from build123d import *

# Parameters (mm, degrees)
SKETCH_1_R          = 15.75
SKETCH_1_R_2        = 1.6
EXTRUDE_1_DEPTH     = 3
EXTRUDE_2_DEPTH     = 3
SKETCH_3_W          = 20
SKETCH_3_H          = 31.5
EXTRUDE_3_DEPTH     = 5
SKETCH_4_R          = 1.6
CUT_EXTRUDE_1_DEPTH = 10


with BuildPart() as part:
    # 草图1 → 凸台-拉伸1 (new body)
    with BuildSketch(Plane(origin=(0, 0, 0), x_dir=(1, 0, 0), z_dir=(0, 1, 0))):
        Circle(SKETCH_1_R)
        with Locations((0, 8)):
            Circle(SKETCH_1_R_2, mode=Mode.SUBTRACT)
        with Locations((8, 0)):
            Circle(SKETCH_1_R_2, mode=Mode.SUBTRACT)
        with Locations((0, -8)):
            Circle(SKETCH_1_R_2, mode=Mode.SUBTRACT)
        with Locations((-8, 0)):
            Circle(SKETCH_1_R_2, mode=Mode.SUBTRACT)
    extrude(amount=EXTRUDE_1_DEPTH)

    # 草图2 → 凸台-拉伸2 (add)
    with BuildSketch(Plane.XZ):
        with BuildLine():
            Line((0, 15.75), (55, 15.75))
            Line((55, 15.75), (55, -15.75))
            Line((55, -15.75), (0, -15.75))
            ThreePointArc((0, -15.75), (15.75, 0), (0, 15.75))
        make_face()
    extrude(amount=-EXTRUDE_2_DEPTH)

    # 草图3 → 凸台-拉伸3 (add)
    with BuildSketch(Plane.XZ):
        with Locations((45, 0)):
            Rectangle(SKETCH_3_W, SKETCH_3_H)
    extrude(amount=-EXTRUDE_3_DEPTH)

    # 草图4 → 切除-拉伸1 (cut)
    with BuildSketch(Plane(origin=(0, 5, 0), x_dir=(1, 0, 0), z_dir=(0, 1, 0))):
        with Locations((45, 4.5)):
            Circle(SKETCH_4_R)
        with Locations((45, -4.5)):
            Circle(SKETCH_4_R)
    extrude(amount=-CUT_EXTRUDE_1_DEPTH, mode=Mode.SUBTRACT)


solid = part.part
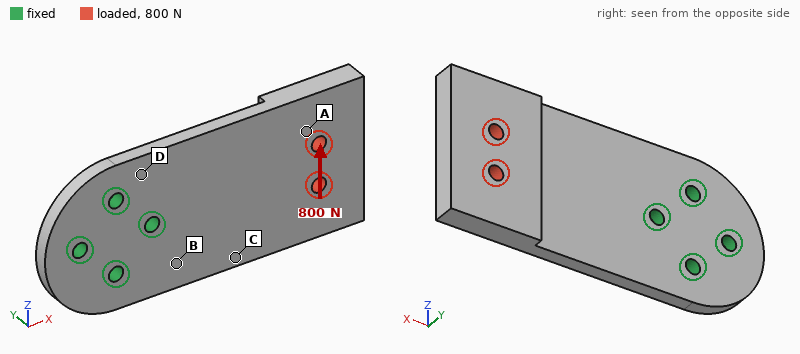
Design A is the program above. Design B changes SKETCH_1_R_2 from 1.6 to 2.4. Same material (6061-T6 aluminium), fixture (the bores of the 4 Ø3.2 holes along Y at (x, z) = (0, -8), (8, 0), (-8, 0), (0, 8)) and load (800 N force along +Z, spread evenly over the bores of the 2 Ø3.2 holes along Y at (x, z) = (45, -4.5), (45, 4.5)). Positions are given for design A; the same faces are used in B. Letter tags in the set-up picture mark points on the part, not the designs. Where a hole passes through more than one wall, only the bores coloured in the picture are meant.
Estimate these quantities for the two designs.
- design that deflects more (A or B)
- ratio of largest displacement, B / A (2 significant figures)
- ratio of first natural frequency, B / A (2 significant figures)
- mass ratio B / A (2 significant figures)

A
0.92
1.0
0.98
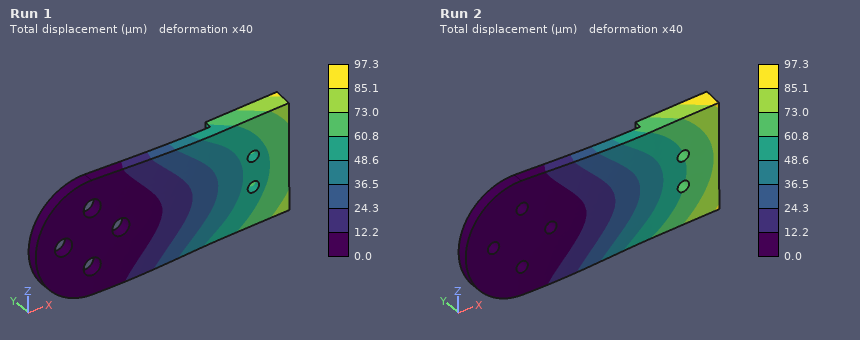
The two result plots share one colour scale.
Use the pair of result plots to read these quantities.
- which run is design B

Run 1
